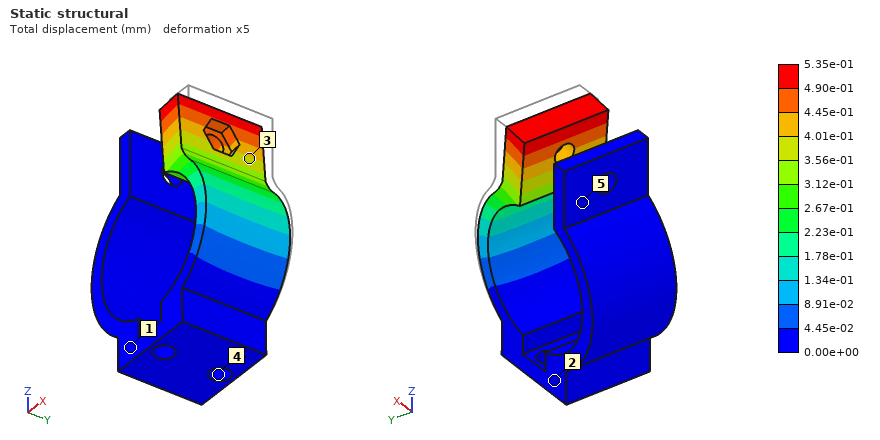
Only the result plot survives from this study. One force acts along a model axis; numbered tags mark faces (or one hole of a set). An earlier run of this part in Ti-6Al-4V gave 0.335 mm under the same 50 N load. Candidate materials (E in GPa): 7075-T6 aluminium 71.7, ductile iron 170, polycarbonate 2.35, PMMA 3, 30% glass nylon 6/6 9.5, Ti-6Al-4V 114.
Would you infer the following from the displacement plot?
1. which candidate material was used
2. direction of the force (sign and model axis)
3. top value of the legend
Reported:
7075-T6 aluminium
-X
5.35e-01 mm
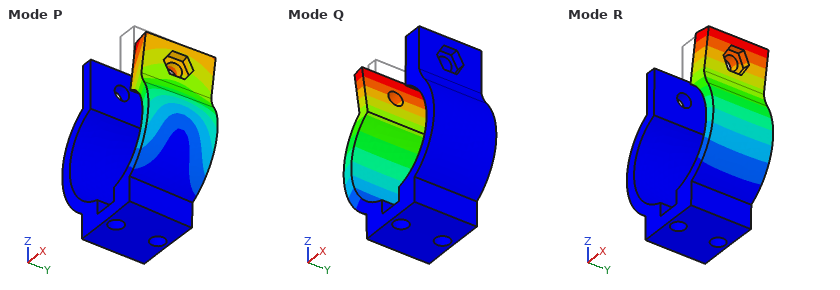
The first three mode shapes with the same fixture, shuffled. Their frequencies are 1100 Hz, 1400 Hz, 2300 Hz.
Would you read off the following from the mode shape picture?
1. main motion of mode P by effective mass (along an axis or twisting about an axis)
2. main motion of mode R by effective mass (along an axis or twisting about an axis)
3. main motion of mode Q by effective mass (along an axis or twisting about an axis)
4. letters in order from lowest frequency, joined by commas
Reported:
along Y
along X
along X
R, Q, P
